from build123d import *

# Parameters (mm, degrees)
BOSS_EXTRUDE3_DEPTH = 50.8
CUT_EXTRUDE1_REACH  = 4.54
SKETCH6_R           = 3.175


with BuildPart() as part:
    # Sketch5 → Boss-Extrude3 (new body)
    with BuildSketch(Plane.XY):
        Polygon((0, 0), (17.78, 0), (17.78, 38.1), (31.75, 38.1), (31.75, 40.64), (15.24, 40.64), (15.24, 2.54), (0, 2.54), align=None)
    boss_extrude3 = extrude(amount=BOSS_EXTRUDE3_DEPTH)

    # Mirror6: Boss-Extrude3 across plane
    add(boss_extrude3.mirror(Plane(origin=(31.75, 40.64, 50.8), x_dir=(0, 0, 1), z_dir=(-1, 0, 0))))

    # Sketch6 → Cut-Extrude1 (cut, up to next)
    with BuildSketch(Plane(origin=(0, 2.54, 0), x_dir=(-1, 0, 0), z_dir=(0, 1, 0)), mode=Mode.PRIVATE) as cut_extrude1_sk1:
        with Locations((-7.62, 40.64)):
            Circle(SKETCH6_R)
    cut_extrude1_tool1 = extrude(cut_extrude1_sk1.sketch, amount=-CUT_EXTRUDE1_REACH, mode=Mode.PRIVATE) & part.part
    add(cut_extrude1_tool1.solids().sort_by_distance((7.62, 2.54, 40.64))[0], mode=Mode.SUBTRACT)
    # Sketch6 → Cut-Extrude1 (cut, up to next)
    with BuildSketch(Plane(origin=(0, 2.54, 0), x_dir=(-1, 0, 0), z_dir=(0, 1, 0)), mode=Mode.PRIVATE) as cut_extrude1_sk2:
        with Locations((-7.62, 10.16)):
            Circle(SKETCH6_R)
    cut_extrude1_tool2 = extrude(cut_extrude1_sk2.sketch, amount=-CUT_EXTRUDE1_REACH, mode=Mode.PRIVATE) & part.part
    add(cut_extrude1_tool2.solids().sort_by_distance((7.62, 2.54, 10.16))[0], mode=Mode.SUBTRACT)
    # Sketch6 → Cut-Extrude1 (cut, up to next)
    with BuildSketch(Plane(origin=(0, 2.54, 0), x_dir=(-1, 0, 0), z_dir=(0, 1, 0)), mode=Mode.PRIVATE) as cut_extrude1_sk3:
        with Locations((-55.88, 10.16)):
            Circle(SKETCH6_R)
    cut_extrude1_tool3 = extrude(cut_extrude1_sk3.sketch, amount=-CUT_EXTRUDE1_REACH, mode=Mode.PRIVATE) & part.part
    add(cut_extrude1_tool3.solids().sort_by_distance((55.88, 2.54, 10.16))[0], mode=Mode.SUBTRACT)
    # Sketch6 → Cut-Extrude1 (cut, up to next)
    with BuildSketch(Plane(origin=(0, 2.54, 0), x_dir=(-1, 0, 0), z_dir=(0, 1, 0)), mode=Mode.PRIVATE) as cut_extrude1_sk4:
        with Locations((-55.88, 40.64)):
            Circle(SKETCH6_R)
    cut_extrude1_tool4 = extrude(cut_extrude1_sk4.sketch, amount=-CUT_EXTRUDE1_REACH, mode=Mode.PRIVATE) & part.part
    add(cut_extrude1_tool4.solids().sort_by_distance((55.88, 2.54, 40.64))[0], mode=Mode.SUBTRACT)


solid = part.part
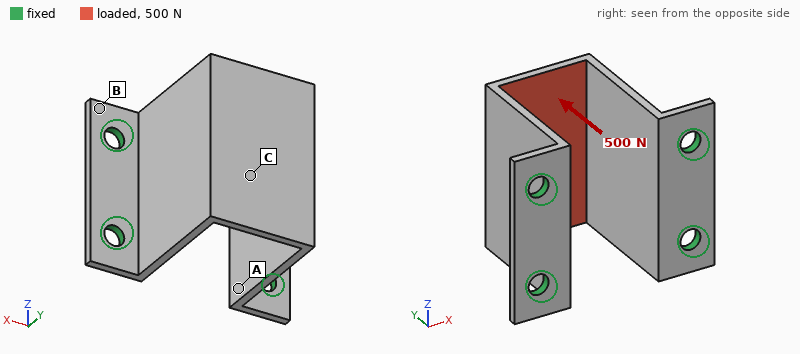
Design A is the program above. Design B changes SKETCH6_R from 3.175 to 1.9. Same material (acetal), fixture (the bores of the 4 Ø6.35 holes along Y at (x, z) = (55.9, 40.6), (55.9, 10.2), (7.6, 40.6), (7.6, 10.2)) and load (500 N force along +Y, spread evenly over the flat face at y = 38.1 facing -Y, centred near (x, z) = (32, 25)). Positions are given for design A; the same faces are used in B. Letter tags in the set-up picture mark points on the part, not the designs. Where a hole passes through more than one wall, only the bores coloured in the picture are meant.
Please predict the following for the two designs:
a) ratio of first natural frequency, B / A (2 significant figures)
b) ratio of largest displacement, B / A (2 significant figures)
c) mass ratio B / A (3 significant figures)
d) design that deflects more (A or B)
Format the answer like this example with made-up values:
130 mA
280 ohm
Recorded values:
0.98
1.1
1.01
B
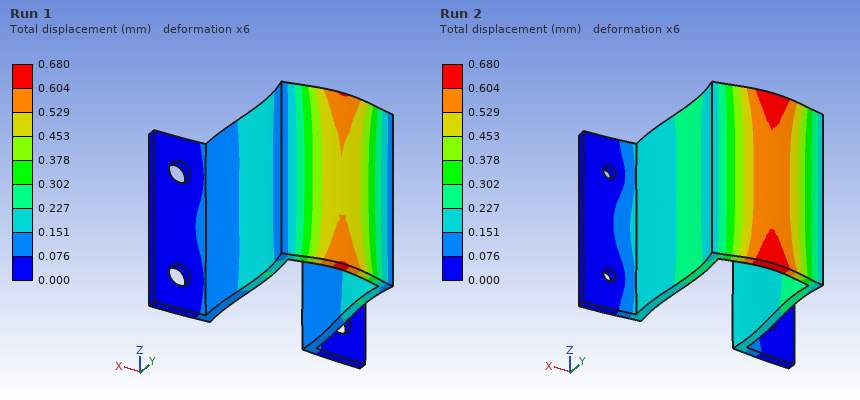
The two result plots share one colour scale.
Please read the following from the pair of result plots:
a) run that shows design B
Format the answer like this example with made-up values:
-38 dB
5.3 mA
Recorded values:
Run 2
